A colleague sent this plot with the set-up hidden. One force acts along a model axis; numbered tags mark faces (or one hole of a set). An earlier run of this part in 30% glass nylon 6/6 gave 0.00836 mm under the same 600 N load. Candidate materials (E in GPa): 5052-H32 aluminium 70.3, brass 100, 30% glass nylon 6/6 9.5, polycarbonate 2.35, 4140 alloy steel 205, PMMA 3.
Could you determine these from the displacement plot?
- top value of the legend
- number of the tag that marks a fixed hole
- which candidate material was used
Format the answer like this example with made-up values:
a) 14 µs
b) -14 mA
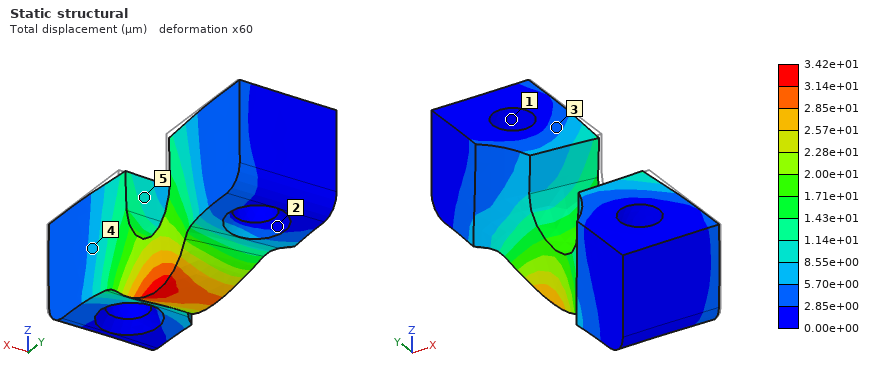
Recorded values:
a) 3.42e+01 µm
b) 1
c) polycarbonate
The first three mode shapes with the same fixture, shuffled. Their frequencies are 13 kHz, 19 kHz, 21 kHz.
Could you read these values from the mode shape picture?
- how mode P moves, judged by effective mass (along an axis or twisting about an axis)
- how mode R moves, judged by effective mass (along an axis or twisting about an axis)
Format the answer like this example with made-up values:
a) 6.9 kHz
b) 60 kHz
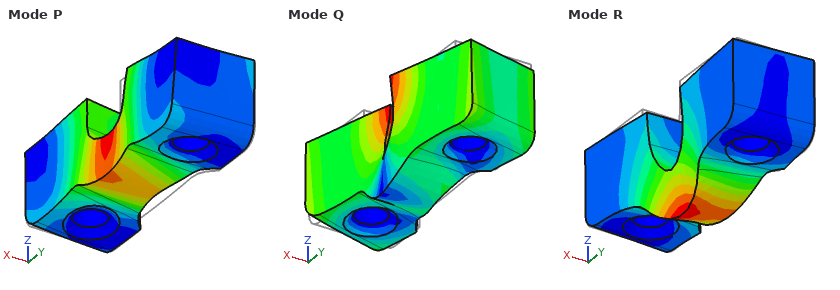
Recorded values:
a) along Z
b) along X
